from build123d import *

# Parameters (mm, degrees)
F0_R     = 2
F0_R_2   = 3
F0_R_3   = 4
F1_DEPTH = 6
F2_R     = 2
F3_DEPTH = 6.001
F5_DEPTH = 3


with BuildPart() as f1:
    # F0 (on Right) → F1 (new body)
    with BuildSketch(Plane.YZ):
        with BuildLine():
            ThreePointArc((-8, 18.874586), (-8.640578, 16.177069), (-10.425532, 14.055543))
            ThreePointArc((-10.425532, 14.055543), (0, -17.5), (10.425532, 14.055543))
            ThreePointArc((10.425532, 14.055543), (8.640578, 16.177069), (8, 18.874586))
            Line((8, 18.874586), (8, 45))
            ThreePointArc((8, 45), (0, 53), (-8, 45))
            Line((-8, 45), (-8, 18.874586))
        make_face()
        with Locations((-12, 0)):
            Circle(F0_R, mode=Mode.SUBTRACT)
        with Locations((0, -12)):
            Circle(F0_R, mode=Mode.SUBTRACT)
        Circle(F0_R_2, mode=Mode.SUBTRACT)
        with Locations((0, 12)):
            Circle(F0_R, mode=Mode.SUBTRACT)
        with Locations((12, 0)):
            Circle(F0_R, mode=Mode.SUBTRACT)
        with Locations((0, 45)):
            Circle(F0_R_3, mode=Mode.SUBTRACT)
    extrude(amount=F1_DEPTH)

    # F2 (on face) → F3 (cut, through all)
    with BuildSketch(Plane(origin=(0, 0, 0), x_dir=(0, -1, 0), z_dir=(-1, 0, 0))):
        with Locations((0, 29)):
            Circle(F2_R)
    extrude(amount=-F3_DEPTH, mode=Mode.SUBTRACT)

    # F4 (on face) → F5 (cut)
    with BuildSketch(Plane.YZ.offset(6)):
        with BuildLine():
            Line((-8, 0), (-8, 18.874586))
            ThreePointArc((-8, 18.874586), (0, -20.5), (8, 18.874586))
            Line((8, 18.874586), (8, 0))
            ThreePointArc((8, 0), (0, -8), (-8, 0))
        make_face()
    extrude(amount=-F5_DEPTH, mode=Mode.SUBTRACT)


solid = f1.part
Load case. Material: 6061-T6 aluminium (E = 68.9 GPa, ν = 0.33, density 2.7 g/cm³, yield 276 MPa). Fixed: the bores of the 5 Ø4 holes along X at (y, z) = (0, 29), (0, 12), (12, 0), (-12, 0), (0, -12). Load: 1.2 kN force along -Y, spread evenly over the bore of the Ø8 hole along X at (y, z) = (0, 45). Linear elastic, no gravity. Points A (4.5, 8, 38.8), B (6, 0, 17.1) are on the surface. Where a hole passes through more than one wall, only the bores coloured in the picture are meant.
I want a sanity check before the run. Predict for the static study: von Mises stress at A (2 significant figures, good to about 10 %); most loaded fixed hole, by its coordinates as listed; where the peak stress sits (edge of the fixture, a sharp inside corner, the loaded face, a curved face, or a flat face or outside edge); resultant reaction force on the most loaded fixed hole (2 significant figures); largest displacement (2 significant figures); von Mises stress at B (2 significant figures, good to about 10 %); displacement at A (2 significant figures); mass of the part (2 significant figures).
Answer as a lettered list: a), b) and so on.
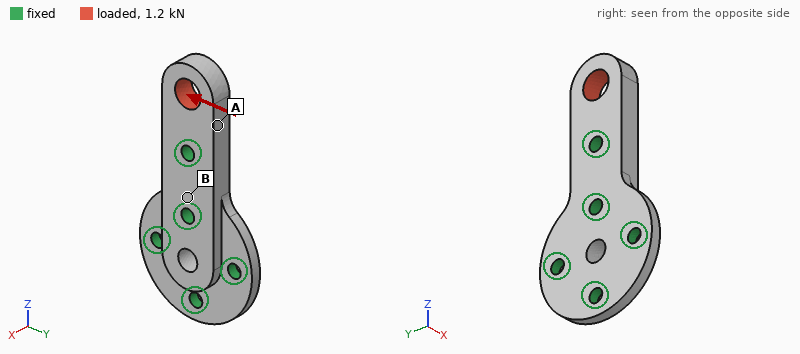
a) 49 MPa
b) (0, 29)
c) edge of the fixture
d) 1.8 kN
e) 58 µm
f) 15 MPa
g) 24 µm
h) 18 g
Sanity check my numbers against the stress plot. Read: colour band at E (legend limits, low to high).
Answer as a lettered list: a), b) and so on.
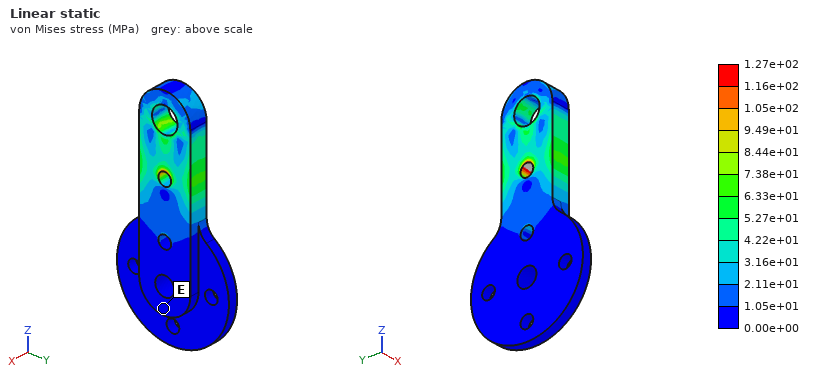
a) 0.00e+00 to 1.05e+01 MPa
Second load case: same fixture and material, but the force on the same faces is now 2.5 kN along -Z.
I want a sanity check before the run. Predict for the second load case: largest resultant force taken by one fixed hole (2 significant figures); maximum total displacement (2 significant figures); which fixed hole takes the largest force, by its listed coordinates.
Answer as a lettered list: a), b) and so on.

a) 2.1 kN
b) 14 µm
c) (0, 29)
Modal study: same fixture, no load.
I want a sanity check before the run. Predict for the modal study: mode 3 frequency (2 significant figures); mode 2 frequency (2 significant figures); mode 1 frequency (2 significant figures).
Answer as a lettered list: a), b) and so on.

a) 22 kHz
b) 16 kHz
c) 10 kHz
